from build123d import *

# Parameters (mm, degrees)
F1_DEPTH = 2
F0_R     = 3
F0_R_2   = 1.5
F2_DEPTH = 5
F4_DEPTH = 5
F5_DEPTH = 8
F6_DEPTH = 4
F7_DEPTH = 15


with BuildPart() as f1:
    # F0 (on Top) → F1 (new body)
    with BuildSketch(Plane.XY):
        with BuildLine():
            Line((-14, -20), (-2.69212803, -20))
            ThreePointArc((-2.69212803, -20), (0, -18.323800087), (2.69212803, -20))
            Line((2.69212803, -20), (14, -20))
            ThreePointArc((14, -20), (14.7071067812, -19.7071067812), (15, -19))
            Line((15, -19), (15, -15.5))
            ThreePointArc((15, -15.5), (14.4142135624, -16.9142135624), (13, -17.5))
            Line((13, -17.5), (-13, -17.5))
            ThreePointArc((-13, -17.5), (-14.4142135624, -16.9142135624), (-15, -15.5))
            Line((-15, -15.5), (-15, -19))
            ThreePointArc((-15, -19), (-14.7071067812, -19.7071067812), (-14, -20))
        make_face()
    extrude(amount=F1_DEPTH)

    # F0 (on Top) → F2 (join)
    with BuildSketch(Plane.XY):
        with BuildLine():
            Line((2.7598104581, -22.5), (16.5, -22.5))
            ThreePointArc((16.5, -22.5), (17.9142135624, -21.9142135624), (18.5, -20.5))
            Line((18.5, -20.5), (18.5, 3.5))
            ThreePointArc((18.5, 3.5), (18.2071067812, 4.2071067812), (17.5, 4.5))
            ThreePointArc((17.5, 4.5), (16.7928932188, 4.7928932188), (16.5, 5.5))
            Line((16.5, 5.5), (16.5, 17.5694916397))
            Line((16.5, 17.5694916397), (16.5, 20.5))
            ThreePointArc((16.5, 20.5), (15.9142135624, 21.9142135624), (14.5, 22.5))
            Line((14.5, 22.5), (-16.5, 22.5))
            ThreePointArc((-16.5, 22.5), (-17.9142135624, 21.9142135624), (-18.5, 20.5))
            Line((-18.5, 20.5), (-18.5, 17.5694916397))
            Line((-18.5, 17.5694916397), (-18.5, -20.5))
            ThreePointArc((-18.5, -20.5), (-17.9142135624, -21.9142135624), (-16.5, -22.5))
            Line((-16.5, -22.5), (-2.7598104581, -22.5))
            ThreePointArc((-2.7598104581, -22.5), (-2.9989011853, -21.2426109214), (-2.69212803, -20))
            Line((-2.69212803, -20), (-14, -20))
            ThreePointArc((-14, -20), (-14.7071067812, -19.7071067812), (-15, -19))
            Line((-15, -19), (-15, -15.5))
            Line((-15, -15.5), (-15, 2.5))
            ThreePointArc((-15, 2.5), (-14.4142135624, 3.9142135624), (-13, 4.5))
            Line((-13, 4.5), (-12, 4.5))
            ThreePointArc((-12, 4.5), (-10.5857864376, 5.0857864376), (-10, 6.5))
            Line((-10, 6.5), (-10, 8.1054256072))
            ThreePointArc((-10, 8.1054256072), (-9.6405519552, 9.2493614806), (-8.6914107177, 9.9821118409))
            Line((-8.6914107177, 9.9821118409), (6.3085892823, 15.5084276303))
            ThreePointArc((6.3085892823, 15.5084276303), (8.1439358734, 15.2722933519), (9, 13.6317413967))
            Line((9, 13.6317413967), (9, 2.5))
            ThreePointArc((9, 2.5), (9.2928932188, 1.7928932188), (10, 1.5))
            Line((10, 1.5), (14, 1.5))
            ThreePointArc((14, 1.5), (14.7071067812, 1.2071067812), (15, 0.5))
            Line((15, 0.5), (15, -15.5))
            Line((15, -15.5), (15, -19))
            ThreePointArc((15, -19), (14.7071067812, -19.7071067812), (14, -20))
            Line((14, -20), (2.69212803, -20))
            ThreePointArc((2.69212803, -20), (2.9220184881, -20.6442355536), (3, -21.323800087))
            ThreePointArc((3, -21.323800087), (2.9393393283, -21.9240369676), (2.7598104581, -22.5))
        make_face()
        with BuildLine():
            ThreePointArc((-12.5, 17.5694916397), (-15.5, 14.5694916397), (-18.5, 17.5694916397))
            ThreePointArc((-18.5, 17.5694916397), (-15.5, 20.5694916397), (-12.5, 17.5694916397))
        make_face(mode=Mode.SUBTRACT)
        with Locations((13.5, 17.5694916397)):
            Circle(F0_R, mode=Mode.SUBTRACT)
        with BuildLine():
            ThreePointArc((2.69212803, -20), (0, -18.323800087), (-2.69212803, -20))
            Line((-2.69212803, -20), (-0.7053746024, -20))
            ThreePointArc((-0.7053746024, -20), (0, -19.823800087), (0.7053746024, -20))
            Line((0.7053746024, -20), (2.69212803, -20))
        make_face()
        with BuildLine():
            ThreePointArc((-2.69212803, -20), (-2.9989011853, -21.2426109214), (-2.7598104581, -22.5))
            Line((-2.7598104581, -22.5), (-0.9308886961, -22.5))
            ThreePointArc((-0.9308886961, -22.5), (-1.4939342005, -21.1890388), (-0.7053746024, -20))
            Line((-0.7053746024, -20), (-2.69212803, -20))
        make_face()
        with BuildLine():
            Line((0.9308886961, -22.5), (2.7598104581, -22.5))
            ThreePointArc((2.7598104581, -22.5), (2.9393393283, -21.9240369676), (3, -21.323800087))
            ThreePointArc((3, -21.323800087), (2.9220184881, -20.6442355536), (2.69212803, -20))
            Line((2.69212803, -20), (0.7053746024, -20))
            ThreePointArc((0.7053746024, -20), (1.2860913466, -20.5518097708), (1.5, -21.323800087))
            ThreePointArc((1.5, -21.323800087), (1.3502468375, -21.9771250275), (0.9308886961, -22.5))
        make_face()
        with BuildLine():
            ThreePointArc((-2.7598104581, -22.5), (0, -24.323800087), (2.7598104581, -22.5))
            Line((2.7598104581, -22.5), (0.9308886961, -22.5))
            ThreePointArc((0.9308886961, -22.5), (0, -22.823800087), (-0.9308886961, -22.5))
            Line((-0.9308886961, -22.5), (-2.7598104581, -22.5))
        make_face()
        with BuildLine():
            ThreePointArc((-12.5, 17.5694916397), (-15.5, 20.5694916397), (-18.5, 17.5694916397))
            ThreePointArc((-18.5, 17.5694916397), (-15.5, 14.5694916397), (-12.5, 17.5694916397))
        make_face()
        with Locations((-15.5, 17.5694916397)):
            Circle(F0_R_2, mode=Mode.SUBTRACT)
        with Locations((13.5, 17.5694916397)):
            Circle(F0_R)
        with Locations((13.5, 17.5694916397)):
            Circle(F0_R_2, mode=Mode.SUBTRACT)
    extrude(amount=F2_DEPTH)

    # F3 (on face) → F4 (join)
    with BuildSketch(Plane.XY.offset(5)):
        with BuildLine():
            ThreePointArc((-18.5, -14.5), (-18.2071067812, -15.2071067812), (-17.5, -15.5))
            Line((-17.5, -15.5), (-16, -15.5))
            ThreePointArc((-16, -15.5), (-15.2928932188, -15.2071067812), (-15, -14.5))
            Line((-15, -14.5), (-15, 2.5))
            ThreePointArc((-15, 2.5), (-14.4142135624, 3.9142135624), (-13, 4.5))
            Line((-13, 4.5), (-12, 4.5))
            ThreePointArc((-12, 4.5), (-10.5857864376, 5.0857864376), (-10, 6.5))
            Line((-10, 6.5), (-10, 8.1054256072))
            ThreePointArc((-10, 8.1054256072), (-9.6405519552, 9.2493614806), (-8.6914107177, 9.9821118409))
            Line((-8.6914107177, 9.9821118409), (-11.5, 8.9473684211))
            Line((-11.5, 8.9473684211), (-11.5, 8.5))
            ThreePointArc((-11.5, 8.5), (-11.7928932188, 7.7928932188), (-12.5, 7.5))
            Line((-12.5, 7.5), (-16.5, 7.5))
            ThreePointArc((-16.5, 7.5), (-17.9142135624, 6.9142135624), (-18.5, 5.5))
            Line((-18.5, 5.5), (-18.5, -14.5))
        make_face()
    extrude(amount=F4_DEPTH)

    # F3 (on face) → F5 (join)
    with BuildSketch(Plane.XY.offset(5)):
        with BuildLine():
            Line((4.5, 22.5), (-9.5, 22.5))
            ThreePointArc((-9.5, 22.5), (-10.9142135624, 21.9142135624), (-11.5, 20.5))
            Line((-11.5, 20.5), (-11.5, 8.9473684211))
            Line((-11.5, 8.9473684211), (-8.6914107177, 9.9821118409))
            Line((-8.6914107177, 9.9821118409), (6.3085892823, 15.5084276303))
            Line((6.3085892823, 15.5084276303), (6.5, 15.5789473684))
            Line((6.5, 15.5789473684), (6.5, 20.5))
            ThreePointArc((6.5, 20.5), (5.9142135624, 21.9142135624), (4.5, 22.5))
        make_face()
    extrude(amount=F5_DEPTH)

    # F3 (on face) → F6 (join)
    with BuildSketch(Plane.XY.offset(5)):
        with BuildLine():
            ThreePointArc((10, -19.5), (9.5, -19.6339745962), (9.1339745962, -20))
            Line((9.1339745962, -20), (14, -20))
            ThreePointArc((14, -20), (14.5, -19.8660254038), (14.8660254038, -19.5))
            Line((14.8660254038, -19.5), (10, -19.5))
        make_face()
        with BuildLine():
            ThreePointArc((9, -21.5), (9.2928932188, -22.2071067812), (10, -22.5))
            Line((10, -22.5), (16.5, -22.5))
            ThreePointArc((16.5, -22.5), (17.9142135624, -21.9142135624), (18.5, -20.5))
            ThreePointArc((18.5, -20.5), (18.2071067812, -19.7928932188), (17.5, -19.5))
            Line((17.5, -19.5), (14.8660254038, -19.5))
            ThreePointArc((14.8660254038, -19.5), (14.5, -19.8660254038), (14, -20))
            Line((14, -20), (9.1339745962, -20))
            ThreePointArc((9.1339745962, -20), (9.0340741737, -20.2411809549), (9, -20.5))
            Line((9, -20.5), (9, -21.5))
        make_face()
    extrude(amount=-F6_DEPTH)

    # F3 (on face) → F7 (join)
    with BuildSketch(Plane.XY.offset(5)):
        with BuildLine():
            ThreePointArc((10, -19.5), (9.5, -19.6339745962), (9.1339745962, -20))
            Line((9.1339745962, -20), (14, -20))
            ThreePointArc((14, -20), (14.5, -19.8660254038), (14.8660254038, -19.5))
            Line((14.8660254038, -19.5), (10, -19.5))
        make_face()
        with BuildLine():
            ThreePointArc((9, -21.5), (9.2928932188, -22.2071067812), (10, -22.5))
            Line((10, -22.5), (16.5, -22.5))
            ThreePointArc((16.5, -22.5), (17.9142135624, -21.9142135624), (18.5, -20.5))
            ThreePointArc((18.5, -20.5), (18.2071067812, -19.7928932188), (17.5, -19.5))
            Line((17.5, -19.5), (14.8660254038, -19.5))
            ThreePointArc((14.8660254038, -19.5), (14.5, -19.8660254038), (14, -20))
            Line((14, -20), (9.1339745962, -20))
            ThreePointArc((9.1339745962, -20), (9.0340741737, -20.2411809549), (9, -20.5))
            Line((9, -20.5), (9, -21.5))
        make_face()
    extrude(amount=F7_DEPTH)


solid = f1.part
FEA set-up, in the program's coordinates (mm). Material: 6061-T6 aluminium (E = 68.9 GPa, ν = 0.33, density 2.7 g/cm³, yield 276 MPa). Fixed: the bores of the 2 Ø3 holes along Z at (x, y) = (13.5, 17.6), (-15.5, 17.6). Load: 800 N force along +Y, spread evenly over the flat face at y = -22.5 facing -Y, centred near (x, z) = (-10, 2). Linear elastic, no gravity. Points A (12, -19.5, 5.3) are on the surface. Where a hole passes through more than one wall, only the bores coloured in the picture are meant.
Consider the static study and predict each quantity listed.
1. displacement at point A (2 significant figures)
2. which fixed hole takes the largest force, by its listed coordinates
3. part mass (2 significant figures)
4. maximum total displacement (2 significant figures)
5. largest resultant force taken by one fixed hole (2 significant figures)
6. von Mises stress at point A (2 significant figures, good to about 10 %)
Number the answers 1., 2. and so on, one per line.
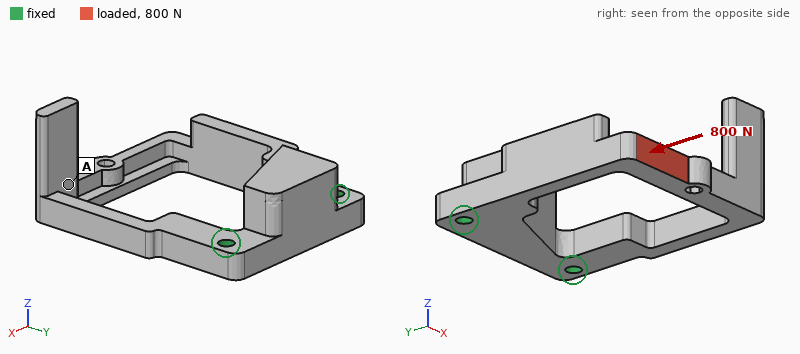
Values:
1. 0.059 mm
2. (-15.5, 17.6)
3. 17 g
4. 0.12 mm
5. 670 N
6. 21 MPa
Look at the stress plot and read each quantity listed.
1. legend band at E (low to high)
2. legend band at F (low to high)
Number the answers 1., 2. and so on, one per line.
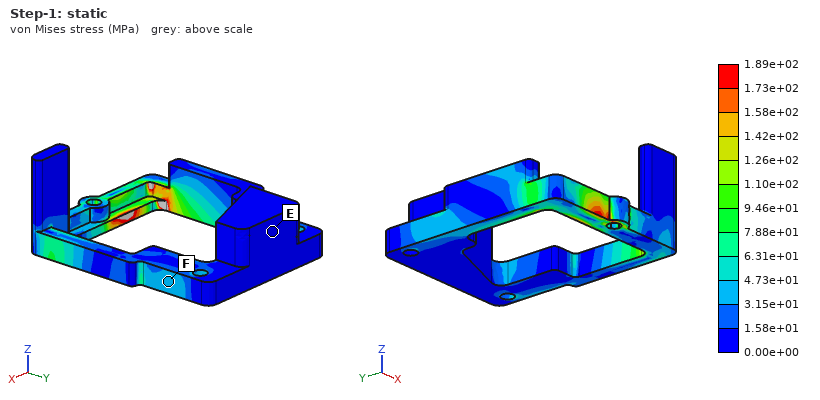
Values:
1. 0.00e+00 to 1.58e+01 MPa
2. 3.15e+01 to 4.73e+01 MPa
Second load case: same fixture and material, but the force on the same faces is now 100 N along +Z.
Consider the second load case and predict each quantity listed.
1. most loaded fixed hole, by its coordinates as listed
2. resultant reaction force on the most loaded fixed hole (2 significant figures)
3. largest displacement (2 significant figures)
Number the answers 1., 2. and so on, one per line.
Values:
1. (-15.5, 17.6)
2. 93 N
3. 0.17 mm
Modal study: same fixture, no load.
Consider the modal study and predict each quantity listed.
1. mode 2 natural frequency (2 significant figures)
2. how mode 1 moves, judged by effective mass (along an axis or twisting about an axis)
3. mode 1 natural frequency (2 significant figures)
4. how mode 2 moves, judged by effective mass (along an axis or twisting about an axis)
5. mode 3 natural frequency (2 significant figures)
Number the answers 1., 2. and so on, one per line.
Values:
1. 2900 Hz
2. along Z
3. 1800 Hz
4. along X
5. 3900 Hz
